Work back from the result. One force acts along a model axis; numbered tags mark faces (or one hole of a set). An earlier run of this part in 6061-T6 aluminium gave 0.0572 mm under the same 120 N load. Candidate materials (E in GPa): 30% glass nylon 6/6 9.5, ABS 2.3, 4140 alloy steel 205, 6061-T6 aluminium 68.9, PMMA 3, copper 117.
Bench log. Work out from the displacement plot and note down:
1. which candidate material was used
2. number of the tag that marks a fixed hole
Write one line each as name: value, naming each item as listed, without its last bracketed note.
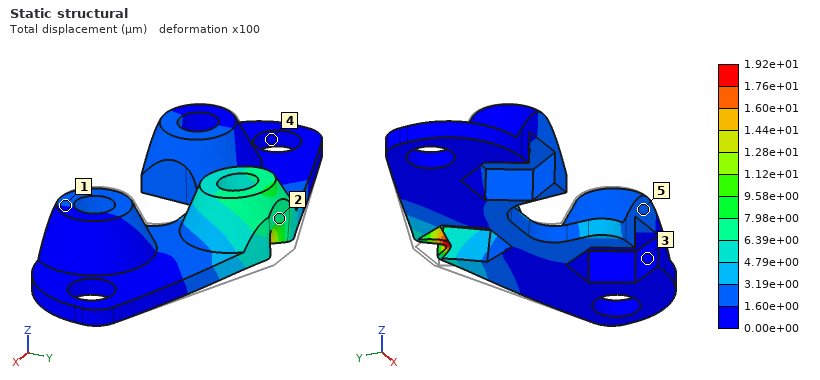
which candidate material was used: 4140 alloy steel
number of the tag that marks a fixed hole: 4
